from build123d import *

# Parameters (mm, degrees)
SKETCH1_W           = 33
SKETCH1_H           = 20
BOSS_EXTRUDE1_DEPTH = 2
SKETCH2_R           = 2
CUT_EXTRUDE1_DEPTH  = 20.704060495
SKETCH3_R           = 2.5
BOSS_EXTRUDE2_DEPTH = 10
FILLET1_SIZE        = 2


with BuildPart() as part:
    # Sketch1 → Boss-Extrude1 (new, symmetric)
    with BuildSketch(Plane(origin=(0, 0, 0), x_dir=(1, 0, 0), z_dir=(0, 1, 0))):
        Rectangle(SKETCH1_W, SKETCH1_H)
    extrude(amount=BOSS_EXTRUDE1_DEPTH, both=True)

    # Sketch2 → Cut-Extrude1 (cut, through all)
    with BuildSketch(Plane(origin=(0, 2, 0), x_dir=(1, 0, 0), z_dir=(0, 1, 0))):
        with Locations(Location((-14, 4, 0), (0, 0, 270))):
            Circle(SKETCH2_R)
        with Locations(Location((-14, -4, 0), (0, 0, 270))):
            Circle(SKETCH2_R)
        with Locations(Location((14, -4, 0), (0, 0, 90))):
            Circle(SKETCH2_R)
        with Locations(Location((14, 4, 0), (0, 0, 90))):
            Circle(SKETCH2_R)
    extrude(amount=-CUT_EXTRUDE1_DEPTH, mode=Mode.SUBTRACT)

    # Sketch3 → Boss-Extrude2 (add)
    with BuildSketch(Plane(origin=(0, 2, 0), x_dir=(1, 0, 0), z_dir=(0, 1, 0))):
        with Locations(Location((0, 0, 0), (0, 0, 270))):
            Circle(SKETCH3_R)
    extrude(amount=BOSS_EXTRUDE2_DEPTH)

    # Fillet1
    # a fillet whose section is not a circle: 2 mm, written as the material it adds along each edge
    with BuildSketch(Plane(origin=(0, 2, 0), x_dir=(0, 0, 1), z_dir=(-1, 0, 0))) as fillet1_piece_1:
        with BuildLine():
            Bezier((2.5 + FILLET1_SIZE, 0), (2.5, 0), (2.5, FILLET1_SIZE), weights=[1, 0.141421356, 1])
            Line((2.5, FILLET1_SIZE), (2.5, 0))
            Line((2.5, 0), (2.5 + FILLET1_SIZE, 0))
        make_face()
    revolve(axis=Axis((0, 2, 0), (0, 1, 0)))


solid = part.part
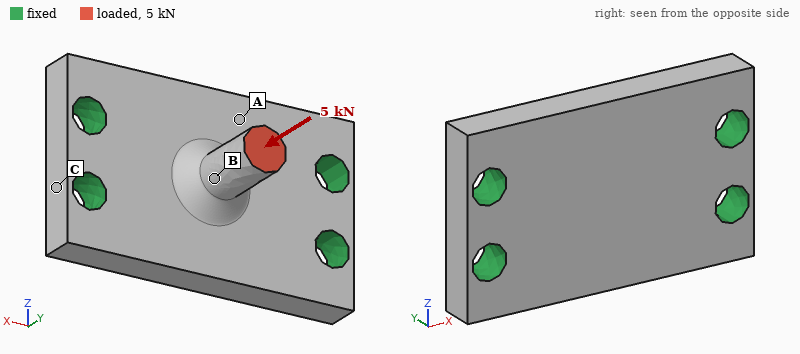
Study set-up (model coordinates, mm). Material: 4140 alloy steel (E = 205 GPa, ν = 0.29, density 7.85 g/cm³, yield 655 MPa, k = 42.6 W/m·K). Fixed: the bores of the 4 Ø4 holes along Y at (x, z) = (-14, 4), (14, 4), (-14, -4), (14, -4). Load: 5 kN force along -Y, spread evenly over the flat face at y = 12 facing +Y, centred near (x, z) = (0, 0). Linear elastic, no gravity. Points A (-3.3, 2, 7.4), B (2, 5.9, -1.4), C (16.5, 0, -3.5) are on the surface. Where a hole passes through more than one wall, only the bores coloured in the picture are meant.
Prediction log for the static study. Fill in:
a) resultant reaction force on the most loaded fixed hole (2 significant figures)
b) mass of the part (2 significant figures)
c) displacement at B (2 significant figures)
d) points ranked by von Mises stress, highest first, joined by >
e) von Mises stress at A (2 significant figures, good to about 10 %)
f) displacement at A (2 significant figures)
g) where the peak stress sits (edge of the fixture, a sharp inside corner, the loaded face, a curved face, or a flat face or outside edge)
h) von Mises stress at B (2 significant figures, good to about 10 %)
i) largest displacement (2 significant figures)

1.3 kN
21 g
26 µm
B > A > C
110 MPa
16 µm
a curved face
240 MPa
33 µm
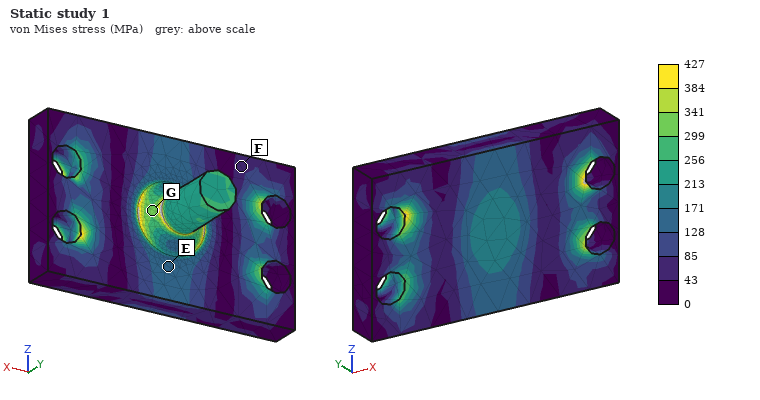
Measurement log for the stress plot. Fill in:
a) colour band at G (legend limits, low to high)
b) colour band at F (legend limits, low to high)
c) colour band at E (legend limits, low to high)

299 to 341 MPa
43 to 85 MPa
128 to 171 MPa
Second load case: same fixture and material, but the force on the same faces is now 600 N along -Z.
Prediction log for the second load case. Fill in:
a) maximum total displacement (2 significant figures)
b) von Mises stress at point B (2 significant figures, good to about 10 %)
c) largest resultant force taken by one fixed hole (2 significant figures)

43 µm
180 MPa
340 N
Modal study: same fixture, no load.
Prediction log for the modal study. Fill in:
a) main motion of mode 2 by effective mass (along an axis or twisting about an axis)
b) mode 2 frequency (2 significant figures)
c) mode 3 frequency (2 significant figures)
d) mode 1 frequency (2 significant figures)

along Y
26 kHz
31 kHz
24 kHz
